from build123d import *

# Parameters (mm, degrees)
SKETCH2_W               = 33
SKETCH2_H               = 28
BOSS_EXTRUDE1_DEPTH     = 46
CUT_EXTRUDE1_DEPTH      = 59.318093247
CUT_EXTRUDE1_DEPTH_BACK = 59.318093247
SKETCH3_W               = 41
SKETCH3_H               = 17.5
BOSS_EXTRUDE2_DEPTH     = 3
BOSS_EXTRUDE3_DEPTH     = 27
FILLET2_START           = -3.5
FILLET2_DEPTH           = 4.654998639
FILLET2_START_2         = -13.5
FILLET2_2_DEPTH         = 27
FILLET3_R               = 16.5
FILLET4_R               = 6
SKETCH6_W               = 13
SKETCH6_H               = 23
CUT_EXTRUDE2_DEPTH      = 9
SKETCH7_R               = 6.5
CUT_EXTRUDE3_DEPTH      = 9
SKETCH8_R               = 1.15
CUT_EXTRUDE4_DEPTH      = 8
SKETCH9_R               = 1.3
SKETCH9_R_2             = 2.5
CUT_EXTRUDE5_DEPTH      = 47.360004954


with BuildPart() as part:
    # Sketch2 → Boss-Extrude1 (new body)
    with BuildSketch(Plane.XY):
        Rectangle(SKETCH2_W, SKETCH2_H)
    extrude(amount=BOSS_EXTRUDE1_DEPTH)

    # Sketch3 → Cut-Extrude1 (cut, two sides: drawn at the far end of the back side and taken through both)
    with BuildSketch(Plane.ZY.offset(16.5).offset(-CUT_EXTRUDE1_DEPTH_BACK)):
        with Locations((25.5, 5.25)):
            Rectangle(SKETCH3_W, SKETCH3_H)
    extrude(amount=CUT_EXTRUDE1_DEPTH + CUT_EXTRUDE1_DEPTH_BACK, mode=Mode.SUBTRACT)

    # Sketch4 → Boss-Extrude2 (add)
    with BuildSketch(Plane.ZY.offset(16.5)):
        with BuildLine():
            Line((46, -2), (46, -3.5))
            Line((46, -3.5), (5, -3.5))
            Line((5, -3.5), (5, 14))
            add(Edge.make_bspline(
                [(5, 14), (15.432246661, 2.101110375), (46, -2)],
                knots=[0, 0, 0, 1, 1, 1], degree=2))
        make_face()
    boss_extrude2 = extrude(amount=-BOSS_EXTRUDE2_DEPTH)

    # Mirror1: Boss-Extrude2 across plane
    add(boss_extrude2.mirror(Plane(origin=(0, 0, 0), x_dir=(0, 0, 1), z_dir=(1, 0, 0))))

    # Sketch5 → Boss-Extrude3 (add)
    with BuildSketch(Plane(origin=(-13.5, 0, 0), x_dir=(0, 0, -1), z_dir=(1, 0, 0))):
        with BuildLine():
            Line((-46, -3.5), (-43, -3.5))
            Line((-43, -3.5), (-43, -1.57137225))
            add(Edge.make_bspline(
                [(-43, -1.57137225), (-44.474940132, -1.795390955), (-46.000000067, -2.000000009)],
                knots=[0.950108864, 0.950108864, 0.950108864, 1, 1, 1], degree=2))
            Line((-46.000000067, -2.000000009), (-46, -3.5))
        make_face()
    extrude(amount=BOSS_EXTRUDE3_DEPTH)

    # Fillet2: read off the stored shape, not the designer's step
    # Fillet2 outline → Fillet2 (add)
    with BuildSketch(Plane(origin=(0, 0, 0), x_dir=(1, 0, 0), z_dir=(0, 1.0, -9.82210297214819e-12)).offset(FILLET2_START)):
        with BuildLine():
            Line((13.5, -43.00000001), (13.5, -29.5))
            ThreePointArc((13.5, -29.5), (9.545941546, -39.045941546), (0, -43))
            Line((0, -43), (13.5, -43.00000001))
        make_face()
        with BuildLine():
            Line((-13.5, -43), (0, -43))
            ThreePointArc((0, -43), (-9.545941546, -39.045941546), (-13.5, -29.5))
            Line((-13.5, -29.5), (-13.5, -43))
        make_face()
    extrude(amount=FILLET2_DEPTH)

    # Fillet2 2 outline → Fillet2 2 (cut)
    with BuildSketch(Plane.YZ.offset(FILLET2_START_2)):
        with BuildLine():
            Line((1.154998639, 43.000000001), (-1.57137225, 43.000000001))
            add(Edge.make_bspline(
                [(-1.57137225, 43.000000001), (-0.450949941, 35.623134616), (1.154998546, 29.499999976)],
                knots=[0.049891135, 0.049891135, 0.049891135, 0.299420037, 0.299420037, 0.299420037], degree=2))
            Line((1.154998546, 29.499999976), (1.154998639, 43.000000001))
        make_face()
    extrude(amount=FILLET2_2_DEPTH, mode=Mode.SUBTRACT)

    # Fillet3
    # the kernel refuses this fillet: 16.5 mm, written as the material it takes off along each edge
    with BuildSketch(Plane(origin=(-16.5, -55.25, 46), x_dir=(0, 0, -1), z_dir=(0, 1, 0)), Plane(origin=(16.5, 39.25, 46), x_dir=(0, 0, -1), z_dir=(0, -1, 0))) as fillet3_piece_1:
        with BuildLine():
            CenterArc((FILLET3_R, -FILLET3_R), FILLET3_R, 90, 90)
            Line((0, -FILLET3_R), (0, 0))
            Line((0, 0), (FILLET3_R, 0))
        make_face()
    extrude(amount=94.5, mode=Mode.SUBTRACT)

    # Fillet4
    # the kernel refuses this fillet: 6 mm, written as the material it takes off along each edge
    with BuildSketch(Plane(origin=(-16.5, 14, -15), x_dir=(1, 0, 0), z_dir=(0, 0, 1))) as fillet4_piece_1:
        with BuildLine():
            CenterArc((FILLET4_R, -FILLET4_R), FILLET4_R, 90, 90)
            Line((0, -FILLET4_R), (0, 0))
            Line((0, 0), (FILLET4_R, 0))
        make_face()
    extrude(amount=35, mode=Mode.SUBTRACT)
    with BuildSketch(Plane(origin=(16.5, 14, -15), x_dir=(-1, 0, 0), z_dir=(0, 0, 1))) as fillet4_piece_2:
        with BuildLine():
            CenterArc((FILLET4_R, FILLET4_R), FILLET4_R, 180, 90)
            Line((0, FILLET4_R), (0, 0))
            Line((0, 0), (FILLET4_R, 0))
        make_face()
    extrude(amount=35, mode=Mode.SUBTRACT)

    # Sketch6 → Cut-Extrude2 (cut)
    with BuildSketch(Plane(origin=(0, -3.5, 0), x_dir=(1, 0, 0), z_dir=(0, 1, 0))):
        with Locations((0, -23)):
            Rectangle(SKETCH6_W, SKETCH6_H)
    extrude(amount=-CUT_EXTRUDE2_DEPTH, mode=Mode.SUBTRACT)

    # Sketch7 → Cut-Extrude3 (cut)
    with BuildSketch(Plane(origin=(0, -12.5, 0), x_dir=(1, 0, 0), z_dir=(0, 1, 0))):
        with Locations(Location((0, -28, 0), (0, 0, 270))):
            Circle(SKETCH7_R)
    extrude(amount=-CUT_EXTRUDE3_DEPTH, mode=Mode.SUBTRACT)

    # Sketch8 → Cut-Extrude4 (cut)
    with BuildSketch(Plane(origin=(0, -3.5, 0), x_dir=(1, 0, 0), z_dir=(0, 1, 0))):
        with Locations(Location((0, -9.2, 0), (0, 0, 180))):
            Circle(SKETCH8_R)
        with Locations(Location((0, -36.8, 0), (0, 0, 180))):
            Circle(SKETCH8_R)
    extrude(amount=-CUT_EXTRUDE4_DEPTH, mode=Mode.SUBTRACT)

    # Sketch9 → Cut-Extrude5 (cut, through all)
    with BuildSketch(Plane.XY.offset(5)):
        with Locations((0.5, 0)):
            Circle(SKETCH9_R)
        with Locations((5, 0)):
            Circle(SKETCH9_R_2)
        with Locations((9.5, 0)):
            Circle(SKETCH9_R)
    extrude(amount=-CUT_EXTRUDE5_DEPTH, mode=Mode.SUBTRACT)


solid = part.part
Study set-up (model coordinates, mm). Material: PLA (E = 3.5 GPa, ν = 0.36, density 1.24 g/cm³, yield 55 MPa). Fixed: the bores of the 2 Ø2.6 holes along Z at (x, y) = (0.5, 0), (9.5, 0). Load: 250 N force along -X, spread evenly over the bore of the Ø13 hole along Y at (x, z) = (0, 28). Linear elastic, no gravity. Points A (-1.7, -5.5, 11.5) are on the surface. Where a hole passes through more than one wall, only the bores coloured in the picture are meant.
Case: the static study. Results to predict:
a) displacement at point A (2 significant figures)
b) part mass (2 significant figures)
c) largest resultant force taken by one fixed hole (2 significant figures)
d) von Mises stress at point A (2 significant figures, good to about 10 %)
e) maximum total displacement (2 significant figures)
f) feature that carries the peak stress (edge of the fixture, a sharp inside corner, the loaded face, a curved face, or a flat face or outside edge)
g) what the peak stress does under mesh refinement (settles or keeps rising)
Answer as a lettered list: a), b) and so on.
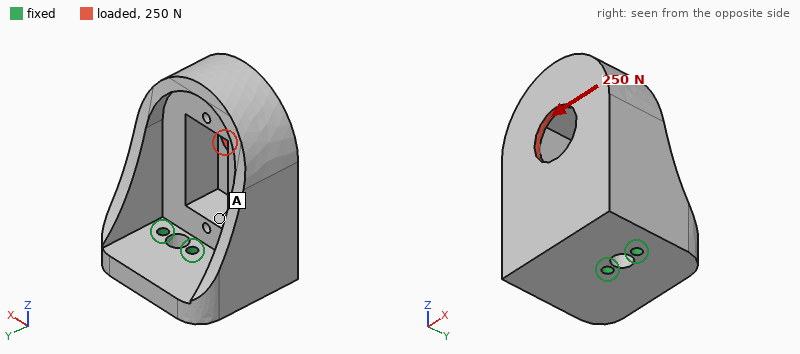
a) 0.12 mm
b) 20 g
c) 540 N
d) 7.3 MPa
e) 0.54 mm
f) edge of the fixture
g) keeps rising
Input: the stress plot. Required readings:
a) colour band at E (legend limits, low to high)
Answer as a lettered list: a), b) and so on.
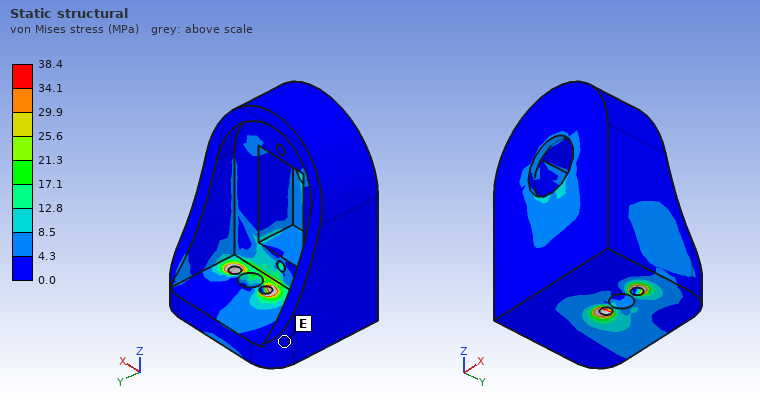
a) 0.0 to 4.3 MPa
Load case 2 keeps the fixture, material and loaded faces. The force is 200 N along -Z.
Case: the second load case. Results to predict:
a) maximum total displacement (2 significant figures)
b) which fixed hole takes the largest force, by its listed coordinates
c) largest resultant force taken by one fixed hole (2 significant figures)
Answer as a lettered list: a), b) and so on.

a) 0.48 mm
b) (0.5, 0)
c) 160 N
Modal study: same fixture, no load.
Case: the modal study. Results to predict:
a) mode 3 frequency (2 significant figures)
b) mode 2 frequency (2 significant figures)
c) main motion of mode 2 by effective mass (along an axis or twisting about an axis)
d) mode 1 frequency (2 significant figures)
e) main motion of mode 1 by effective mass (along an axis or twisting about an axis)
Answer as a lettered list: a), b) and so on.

a) 2500 Hz
b) 1100 Hz
c) along X
d) 770 Hz
e) along Y
